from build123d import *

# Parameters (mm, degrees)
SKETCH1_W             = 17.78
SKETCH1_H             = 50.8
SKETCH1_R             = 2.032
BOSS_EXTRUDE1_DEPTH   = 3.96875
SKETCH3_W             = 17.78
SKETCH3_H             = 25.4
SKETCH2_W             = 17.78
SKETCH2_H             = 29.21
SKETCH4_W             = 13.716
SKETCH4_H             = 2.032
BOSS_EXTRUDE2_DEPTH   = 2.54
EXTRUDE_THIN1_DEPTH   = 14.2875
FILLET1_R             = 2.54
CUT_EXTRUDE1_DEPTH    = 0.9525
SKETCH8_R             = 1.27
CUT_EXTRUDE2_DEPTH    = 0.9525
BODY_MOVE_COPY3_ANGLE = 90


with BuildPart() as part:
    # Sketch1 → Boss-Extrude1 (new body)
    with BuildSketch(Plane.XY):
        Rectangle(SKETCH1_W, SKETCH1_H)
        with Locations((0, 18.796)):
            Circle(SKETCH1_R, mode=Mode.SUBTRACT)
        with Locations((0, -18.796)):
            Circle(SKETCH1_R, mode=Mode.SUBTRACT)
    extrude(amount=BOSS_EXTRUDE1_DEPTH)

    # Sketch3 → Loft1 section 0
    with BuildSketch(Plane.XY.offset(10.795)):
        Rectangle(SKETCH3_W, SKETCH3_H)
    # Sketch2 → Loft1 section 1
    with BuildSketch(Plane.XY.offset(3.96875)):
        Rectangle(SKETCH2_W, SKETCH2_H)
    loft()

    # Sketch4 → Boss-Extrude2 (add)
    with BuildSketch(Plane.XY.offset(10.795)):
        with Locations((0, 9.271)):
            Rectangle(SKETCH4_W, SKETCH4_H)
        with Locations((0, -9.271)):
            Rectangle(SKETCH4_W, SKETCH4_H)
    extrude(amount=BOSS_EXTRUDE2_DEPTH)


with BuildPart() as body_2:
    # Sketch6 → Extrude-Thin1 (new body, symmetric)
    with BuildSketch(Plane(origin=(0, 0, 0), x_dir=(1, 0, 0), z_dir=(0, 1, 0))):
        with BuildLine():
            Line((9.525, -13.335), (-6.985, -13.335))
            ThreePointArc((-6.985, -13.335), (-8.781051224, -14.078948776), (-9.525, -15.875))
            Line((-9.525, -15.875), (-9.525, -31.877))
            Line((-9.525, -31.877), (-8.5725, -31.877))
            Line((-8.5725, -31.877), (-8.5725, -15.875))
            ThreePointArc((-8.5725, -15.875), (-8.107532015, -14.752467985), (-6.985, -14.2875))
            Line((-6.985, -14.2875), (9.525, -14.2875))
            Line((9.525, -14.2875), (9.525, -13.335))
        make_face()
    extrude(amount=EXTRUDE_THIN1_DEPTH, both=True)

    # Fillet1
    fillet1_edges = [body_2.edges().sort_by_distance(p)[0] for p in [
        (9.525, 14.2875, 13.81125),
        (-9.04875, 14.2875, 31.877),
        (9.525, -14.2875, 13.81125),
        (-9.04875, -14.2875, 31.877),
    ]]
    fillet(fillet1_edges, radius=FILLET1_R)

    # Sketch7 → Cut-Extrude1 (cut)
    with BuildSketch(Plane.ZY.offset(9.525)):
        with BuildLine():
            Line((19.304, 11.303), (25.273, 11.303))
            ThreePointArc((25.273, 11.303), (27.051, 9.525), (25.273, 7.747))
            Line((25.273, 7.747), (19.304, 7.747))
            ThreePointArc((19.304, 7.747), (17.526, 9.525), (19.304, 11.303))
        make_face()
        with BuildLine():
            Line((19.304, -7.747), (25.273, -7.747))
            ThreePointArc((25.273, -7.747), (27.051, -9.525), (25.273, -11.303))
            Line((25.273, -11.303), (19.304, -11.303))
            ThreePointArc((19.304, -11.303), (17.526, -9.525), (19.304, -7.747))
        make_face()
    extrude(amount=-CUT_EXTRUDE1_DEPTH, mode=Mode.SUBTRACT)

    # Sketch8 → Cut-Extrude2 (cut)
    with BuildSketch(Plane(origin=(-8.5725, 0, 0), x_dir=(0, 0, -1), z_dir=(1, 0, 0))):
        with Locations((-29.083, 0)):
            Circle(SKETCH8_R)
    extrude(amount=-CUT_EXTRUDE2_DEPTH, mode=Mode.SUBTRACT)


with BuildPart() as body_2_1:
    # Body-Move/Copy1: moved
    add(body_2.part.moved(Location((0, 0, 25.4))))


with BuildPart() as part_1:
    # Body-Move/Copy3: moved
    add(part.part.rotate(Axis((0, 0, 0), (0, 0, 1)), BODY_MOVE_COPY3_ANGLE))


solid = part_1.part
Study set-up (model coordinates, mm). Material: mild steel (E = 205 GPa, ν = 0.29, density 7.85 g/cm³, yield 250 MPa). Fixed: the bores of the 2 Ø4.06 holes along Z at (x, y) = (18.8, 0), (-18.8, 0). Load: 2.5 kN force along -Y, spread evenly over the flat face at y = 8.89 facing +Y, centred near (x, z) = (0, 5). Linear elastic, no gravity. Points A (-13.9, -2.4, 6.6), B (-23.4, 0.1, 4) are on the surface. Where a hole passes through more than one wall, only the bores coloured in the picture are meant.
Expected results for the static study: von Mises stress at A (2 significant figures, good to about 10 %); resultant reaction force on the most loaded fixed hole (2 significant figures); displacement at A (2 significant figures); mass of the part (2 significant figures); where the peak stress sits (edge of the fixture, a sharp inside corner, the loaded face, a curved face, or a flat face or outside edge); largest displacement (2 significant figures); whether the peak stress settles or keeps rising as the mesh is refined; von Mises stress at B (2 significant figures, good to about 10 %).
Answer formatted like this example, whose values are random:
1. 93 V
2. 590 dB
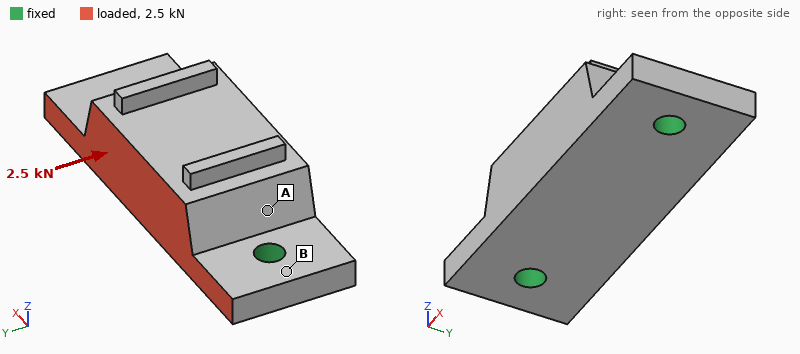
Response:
1. 26 MPa
2. 1.3 kN
3. 4.4 µm
4. 54 g
5. edge of the fixture
6. 9.4 µm
7. keeps rising
8. 12 MPa
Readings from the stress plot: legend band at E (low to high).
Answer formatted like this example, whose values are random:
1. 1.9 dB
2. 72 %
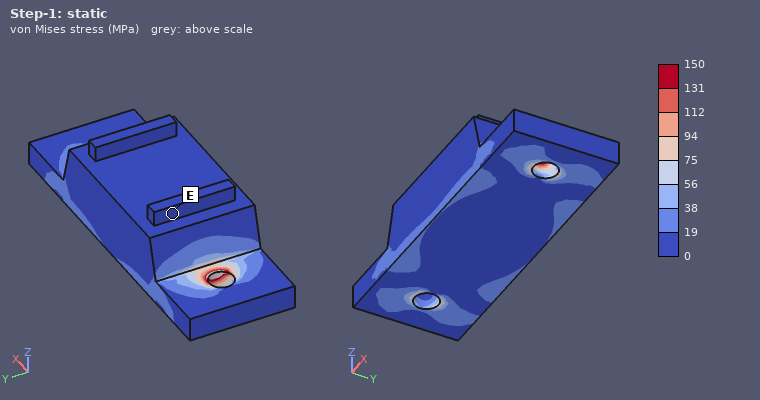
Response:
1. 0 to 19 MPa
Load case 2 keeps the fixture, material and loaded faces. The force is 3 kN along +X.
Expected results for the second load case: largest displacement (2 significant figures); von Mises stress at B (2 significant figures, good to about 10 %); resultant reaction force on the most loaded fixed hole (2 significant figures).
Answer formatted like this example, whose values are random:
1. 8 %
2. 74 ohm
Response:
1. 2.8 µm
2. 13 MPa
3. 1.7 kN
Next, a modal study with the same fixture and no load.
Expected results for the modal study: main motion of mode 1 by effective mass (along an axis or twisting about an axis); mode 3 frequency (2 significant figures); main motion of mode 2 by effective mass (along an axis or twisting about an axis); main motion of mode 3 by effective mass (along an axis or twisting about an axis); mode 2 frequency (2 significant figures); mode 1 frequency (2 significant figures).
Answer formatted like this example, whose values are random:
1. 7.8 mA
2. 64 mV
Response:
1. along Y
2. 25 kHz
3. along Z
4. along Y
5. 17 kHz
6. 11 kHz
